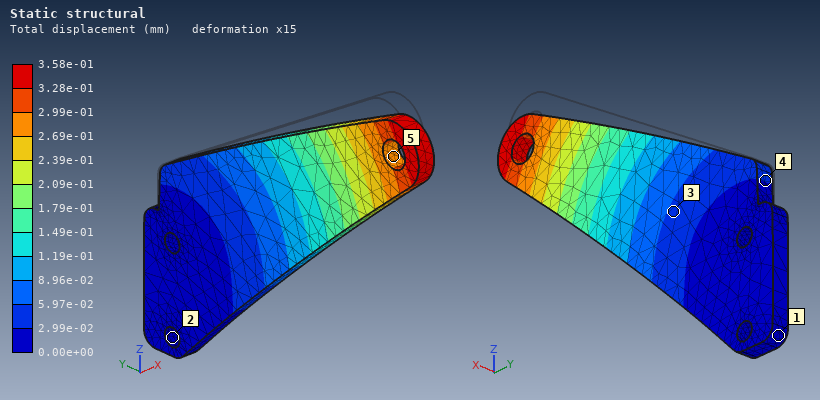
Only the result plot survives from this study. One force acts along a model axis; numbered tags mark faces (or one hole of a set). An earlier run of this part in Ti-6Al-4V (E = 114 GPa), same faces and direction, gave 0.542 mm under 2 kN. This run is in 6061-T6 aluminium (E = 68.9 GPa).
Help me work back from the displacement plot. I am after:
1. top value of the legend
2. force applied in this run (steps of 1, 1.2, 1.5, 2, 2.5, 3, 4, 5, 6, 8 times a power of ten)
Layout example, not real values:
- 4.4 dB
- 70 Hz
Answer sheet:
- 3.58e-01 mm
- 800 N
